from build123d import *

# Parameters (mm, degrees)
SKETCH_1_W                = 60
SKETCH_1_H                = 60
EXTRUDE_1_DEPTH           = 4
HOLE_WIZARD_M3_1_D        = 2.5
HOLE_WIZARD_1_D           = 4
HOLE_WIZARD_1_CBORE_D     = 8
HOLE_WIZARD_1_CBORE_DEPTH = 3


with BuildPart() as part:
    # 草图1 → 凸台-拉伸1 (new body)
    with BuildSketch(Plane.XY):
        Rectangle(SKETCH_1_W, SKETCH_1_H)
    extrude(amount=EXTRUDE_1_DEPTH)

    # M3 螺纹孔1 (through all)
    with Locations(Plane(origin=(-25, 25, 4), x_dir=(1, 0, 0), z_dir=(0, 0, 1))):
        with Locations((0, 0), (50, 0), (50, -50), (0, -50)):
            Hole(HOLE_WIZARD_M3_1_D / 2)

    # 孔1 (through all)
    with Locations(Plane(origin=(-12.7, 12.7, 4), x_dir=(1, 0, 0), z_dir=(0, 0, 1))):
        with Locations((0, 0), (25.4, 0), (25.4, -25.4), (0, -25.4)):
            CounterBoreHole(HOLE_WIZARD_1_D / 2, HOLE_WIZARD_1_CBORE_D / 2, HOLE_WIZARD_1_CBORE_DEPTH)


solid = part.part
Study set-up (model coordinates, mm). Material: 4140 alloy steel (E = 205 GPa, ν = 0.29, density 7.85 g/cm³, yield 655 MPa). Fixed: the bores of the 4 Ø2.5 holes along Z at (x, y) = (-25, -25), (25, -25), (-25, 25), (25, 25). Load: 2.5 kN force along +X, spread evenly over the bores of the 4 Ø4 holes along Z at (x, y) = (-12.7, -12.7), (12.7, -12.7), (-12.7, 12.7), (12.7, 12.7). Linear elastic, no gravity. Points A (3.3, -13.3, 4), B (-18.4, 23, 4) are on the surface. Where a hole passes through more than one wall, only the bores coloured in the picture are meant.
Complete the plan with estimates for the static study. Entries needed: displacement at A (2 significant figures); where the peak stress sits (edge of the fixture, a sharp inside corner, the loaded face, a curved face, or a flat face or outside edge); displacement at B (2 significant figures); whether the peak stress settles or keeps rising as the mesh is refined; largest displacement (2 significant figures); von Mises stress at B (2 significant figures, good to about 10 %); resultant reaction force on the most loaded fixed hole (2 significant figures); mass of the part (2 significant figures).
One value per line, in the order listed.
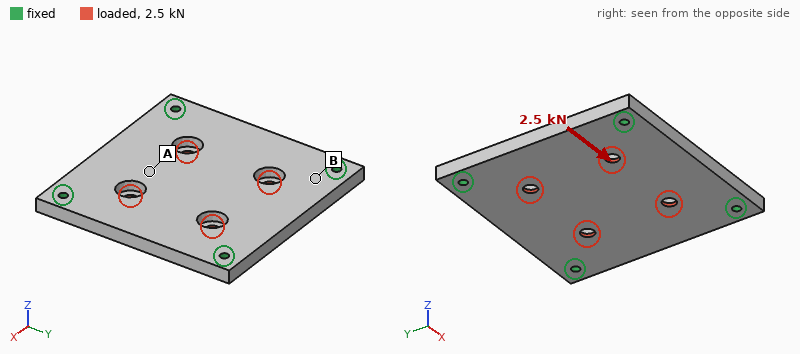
1.4 µm
a sharp inside corner
0.57 µm
keeps rising
2.7 µm
12 MPa
670 N
110 g
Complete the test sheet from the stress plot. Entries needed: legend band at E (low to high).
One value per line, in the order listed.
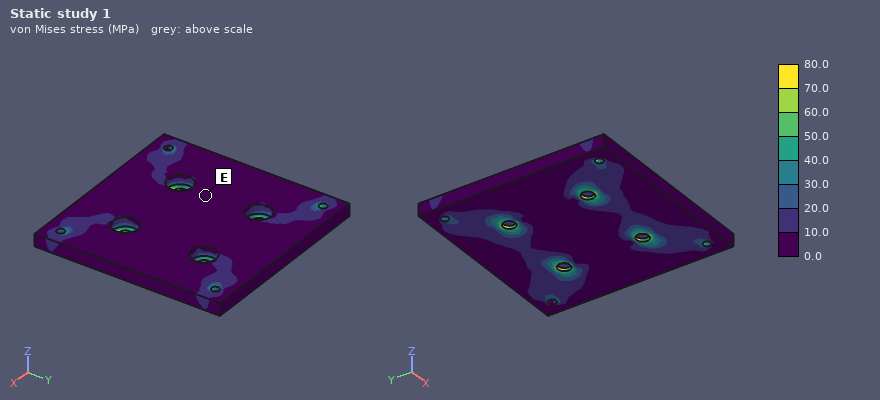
0.0 to 10.0 MPa
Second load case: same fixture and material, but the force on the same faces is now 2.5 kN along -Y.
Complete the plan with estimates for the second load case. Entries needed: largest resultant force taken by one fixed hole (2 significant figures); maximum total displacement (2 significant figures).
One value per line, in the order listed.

670 N
2.7 µm
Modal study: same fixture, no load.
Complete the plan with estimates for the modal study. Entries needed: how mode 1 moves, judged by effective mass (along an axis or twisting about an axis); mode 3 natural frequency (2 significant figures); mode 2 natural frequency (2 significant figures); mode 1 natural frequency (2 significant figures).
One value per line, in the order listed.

along Z
8500 Hz
8500 Hz
5100 Hz
